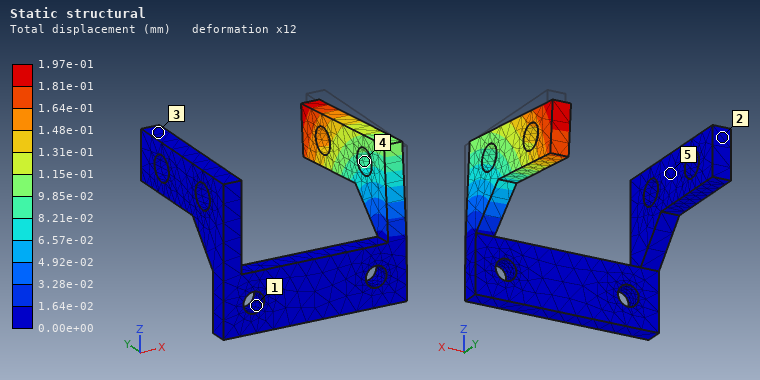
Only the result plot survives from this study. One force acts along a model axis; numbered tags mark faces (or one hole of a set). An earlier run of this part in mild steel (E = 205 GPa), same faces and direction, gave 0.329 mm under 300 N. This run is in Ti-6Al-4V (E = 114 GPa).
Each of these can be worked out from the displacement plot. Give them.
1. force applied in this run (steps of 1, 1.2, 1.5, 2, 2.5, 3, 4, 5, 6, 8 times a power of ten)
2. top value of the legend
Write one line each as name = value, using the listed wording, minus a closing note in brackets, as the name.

force applied in this run = 100 N
top value of the legend = 1.97e-01 mm
